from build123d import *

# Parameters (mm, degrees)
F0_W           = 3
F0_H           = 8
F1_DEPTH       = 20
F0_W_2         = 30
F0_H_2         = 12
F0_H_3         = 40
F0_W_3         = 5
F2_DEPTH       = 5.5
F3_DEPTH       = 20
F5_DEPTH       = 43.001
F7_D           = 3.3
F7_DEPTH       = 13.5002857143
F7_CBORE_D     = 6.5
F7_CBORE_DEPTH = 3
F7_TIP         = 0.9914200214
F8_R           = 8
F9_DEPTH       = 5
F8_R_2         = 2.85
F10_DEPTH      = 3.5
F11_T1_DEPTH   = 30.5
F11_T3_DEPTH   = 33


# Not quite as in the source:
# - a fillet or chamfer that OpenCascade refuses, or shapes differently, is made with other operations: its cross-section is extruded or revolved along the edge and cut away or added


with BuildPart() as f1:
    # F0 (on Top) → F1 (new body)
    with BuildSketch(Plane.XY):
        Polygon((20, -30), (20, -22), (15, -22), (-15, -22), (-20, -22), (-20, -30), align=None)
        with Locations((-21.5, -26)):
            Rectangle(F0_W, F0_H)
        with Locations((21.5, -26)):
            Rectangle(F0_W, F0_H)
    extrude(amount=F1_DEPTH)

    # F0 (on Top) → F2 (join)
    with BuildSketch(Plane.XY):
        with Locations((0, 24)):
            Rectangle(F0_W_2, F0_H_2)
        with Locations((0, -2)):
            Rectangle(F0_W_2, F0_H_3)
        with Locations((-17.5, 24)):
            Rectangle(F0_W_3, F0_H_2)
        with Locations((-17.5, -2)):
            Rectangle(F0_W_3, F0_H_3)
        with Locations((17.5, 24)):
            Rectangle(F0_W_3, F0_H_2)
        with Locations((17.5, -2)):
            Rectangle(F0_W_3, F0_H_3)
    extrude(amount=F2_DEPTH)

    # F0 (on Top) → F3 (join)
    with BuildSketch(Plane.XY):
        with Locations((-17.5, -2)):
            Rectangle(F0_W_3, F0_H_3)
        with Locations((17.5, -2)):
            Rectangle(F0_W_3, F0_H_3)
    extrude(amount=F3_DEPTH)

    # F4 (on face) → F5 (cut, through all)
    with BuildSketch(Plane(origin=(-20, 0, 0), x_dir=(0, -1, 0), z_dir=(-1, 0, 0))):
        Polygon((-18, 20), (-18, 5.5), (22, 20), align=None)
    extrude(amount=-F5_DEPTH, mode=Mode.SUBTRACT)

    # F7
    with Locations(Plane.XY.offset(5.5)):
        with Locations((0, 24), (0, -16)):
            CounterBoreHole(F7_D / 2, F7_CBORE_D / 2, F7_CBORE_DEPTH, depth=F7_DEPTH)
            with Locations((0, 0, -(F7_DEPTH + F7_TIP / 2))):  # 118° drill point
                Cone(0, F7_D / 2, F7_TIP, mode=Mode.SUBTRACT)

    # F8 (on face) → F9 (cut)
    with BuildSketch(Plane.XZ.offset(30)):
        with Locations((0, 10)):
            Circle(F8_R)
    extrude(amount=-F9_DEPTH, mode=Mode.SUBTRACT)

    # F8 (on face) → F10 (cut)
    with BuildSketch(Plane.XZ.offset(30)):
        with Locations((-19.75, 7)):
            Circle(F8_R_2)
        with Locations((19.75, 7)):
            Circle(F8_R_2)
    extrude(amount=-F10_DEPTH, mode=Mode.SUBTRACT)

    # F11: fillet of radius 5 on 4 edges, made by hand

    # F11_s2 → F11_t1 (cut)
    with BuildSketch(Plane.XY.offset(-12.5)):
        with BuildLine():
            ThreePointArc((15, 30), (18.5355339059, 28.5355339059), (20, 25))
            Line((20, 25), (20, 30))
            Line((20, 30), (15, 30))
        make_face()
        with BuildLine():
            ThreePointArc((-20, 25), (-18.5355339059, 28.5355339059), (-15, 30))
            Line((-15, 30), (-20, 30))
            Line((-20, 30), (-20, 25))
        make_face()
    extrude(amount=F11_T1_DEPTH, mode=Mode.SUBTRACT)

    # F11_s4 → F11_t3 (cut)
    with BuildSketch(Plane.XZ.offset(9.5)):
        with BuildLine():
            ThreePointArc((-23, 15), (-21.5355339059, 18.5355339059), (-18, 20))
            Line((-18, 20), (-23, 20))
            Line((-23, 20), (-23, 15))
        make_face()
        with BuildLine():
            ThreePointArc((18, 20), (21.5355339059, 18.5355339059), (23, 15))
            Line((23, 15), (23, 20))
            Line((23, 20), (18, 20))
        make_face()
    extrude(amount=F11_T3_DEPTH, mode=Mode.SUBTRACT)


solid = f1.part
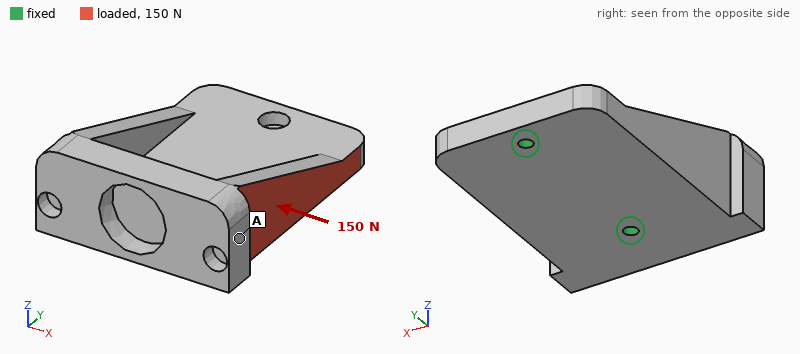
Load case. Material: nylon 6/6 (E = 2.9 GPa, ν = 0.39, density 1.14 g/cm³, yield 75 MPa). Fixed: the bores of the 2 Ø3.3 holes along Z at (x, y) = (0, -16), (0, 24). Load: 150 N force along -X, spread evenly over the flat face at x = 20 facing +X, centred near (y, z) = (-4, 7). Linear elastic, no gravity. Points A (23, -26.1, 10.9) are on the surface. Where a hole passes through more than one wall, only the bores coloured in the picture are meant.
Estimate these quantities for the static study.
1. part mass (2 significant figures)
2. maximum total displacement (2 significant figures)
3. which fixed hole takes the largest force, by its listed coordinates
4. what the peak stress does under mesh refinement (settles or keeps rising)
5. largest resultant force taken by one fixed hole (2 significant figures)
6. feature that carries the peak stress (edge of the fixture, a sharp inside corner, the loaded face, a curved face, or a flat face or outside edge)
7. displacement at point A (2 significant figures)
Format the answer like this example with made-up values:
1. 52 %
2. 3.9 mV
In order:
1. 23 g
2. 0.28 mm
3. (0, -16)
4. keeps rising
5. 100 N
6. edge of the fixture
7. 0.25 mm
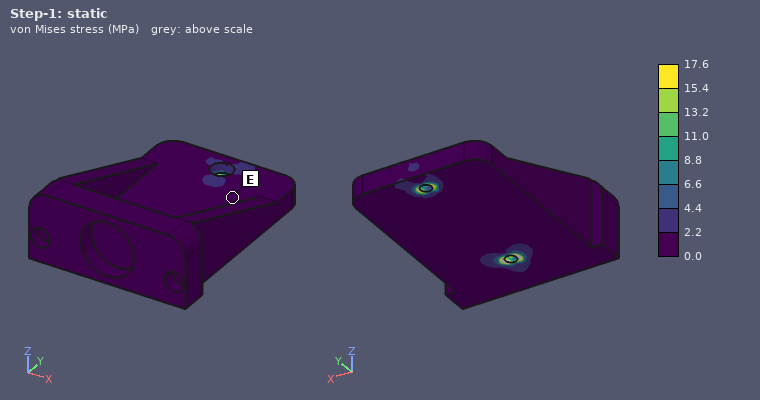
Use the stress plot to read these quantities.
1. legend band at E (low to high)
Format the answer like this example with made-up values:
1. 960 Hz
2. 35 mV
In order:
1. 0.0 to 2.2 MPa
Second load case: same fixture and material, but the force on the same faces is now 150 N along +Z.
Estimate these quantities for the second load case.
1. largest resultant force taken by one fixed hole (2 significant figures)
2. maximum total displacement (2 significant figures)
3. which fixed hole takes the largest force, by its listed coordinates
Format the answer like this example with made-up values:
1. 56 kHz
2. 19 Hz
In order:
1. 110 N
2. 0.92 mm
3. (0, -16)
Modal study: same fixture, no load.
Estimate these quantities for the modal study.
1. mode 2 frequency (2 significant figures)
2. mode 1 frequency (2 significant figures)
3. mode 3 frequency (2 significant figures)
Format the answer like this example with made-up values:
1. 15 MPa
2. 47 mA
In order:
1. 2000 Hz
2. 670 Hz
3. 2200 Hz
